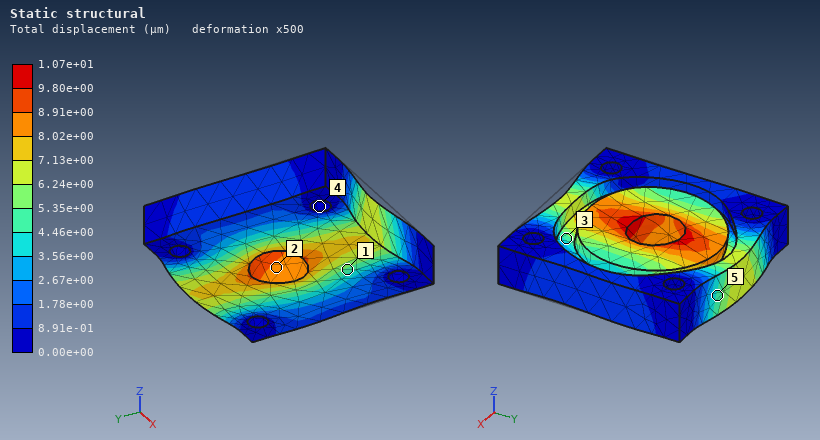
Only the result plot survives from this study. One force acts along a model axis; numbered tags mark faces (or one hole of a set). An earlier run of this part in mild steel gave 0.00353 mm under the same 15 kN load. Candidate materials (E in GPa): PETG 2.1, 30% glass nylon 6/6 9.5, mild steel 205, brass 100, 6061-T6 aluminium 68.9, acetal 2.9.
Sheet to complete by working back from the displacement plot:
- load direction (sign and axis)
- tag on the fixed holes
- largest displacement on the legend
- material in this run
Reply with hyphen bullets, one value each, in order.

- +Y
- 4
- 1.07e+01 µm
- 6061-T6 aluminium
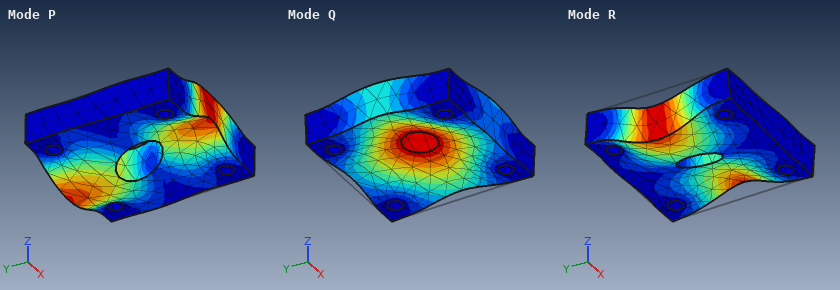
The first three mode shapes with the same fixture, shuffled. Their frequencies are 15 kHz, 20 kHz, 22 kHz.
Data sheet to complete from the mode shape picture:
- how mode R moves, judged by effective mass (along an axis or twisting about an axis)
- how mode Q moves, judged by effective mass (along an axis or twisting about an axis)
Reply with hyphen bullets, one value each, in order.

- twisting about Y
- along Z
